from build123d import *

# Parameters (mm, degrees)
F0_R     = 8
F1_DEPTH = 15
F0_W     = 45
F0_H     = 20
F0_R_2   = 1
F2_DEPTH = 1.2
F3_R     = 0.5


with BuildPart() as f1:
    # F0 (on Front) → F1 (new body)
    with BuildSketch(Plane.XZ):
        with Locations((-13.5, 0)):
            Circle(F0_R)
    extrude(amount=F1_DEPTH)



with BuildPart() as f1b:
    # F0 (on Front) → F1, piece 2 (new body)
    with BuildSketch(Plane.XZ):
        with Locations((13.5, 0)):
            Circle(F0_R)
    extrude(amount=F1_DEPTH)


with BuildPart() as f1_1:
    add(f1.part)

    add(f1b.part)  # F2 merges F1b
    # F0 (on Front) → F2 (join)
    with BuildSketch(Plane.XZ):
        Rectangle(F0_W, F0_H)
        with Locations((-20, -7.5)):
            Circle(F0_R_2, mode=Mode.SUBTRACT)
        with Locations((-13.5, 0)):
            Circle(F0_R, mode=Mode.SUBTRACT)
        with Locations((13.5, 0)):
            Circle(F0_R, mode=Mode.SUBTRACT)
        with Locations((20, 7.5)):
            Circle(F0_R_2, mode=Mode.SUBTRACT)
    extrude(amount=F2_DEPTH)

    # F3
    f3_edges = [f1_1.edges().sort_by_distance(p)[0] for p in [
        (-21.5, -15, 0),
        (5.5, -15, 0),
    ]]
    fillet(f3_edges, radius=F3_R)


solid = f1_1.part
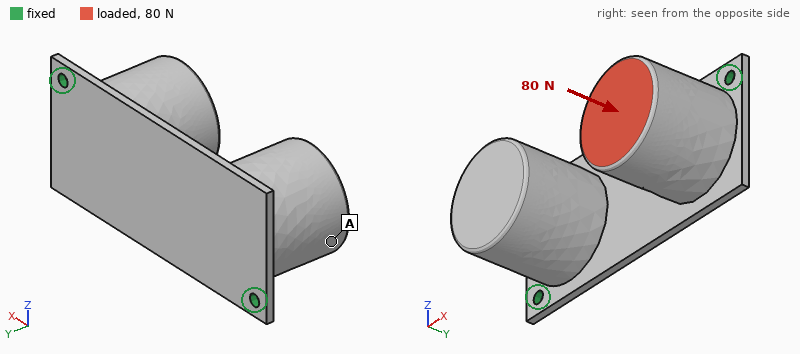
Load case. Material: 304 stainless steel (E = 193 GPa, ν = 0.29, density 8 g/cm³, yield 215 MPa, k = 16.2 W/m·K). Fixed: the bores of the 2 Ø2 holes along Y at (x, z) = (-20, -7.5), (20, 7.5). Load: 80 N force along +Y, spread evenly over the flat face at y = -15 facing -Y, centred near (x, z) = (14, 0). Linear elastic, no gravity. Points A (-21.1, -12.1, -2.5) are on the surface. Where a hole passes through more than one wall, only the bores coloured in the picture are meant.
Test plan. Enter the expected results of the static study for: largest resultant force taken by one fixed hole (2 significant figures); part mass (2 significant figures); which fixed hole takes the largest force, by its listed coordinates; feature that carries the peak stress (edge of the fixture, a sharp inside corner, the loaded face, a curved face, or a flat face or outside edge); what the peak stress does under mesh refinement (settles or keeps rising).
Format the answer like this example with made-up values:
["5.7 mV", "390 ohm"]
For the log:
["64 N", "53 g", "(20, 7.5)", "edge of the fixture", "keeps rising"]
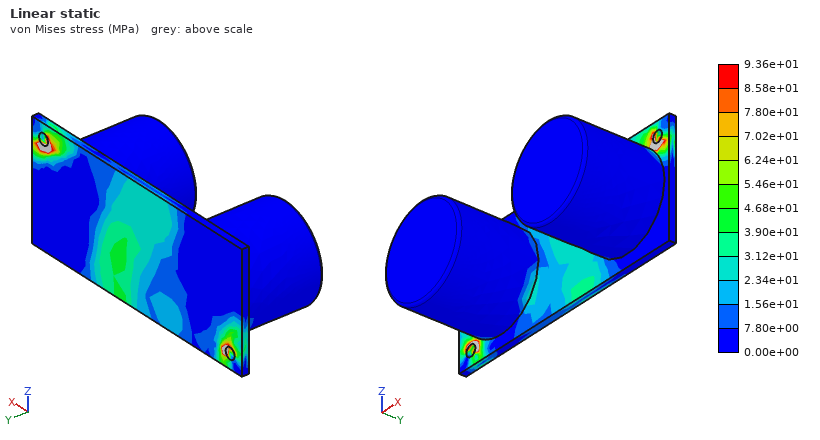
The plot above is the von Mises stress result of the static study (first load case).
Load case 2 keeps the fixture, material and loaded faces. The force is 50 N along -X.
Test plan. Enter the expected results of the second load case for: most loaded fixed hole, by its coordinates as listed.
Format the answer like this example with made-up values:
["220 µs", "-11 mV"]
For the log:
["(20, 7.5)"]
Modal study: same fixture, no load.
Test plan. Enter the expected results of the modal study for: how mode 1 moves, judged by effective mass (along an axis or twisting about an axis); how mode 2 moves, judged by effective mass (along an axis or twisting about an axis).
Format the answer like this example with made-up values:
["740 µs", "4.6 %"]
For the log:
["along Y", "along Z"]
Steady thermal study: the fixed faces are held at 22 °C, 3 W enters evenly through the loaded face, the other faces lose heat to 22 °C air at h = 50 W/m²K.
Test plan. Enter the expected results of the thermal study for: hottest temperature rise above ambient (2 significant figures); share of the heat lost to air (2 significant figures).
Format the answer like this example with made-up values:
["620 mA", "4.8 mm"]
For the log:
["33 K", "64 %"]
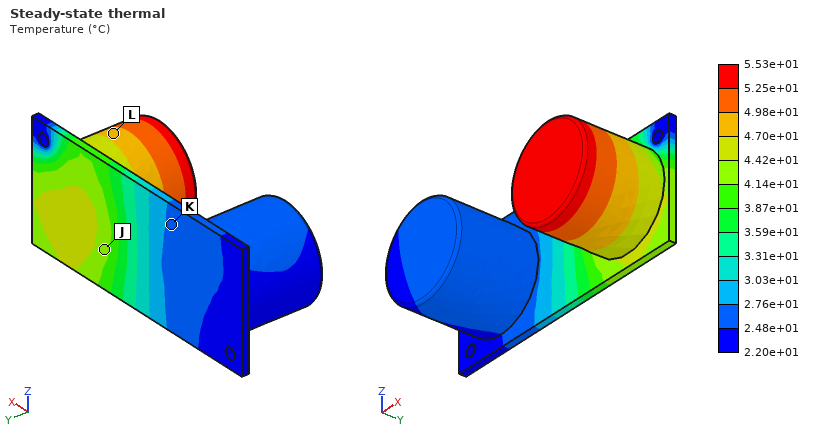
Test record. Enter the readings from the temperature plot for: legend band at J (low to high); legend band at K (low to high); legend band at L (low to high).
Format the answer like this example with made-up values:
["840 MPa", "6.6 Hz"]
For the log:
["4.14e+01 to 4.42e+01 °C", "2.48e+01 to 2.76e+01 °C", "4.70e+01 to 4.98e+01 °C"]
